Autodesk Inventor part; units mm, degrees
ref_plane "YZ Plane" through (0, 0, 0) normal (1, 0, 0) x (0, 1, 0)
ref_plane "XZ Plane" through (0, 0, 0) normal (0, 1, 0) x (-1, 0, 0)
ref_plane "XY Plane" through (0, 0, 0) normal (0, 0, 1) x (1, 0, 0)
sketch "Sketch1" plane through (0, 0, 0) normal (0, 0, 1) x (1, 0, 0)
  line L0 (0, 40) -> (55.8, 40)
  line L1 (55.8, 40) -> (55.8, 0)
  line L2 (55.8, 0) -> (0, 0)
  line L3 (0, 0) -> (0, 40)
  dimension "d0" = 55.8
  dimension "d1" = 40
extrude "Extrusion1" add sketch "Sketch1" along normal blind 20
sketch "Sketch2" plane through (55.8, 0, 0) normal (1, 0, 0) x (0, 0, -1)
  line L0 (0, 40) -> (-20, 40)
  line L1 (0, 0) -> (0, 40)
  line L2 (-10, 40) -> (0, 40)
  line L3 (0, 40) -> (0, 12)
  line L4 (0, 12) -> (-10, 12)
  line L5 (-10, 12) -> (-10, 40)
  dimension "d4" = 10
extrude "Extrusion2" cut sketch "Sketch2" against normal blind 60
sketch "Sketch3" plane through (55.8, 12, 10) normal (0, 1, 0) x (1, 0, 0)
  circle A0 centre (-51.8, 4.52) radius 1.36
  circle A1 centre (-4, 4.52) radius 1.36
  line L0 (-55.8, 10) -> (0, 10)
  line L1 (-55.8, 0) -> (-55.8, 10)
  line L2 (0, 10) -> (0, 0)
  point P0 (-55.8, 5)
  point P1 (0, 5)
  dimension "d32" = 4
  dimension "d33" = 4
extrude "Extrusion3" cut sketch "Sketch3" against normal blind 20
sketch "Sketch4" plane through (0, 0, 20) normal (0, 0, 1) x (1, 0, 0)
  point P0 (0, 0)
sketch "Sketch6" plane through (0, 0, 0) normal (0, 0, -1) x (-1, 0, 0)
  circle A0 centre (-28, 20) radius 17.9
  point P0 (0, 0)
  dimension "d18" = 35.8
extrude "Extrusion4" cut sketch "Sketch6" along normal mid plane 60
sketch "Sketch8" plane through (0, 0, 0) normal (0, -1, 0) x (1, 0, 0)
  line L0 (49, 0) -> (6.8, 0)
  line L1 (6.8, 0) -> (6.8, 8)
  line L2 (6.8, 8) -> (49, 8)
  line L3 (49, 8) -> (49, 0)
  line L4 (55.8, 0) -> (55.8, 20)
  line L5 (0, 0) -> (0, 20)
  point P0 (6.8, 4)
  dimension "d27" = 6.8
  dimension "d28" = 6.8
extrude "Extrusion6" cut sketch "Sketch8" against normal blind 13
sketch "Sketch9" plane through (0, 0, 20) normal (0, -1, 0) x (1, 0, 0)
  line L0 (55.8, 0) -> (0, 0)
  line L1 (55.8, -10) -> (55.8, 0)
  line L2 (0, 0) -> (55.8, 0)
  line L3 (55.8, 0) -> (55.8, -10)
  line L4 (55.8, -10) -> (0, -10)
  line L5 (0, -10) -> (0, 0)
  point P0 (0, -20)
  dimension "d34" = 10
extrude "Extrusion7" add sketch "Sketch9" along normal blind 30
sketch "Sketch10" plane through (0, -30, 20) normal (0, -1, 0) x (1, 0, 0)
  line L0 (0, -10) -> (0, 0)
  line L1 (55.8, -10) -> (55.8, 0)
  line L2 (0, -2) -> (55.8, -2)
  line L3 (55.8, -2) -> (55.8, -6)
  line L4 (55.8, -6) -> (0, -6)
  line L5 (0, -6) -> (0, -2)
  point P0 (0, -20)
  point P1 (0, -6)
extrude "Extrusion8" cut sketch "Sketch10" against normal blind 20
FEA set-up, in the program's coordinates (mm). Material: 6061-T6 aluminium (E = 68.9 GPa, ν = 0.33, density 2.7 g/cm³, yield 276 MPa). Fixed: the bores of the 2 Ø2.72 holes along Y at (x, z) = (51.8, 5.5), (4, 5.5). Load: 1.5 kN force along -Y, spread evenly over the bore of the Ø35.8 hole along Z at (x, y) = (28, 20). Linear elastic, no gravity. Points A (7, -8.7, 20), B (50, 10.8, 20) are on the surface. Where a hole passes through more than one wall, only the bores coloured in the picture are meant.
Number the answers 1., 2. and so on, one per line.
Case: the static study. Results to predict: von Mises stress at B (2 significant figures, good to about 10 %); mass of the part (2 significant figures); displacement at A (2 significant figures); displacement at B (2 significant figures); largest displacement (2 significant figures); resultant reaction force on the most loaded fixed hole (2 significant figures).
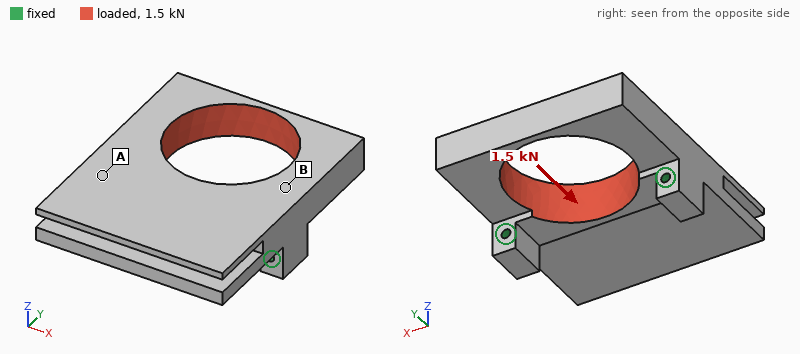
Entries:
1. 6.2 MPa
2. 72 g
3. 10 µm
4. 8.2 µm
5. 25 µm
6. 750 N
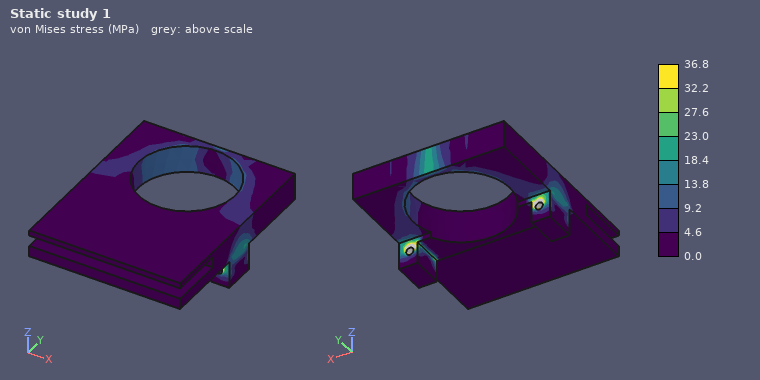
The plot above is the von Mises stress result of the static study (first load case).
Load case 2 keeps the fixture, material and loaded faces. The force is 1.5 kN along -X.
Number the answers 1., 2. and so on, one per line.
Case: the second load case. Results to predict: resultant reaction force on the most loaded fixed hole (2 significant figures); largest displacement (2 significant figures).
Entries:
1. 850 N
2. 37 µm
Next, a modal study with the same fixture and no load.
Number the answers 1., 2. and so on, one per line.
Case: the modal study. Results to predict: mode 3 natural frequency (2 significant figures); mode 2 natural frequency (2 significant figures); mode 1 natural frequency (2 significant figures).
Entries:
1. 4800 Hz
2. 4300 Hz
3. 3100 Hz
